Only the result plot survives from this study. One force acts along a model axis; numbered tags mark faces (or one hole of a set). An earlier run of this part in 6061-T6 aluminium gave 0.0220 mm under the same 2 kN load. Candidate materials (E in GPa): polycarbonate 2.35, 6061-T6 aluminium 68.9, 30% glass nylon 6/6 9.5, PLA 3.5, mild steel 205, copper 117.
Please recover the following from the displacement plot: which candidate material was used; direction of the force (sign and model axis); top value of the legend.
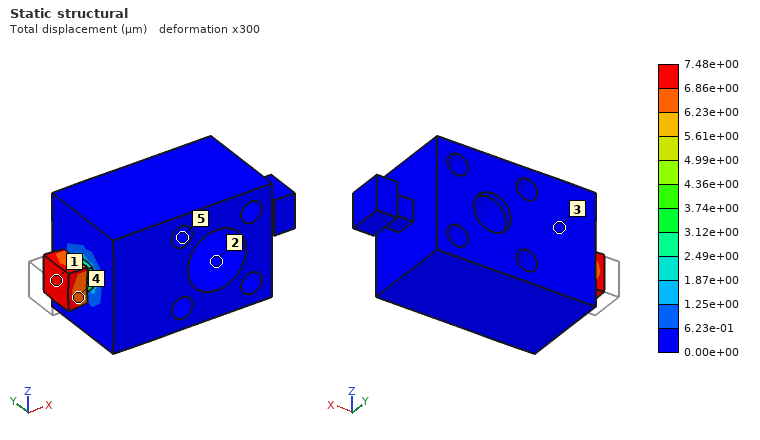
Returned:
mild steel
+X
7.48e+00 µm
